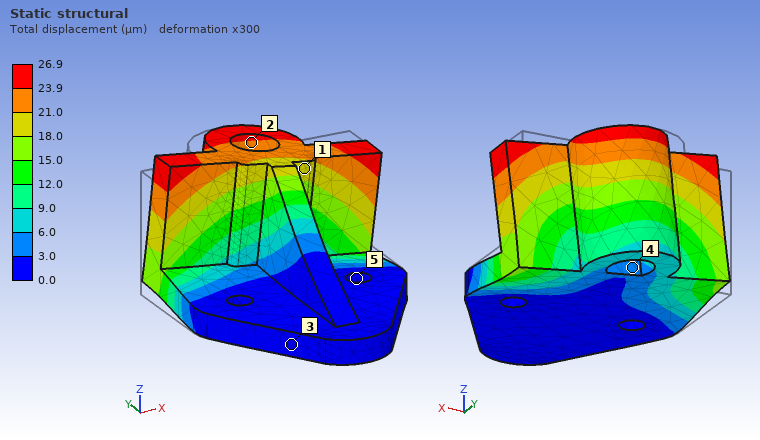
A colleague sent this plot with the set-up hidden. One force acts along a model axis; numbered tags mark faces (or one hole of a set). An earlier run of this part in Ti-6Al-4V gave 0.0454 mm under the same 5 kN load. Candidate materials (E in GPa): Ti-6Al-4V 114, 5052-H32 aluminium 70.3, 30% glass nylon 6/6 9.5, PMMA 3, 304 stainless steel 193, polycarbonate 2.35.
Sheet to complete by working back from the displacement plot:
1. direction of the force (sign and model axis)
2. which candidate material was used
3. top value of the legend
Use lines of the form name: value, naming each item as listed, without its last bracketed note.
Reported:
direction of the force: +X
which candidate material was used: 304 stainless steel
top value of the legend: 26.9 µm
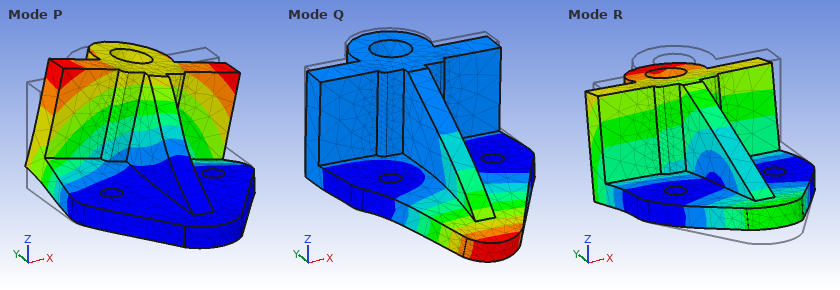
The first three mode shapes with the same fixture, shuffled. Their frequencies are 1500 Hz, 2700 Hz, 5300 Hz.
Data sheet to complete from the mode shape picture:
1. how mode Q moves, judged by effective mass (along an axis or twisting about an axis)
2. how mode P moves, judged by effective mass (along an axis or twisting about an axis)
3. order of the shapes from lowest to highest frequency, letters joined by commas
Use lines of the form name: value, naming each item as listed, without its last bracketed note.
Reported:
how mode Q moves, judged by effective mass: along Z
how mode P moves, judged by effective mass: along X
order of the shapes from lowest to highest frequency, letters joined by commas: R, P, Q
